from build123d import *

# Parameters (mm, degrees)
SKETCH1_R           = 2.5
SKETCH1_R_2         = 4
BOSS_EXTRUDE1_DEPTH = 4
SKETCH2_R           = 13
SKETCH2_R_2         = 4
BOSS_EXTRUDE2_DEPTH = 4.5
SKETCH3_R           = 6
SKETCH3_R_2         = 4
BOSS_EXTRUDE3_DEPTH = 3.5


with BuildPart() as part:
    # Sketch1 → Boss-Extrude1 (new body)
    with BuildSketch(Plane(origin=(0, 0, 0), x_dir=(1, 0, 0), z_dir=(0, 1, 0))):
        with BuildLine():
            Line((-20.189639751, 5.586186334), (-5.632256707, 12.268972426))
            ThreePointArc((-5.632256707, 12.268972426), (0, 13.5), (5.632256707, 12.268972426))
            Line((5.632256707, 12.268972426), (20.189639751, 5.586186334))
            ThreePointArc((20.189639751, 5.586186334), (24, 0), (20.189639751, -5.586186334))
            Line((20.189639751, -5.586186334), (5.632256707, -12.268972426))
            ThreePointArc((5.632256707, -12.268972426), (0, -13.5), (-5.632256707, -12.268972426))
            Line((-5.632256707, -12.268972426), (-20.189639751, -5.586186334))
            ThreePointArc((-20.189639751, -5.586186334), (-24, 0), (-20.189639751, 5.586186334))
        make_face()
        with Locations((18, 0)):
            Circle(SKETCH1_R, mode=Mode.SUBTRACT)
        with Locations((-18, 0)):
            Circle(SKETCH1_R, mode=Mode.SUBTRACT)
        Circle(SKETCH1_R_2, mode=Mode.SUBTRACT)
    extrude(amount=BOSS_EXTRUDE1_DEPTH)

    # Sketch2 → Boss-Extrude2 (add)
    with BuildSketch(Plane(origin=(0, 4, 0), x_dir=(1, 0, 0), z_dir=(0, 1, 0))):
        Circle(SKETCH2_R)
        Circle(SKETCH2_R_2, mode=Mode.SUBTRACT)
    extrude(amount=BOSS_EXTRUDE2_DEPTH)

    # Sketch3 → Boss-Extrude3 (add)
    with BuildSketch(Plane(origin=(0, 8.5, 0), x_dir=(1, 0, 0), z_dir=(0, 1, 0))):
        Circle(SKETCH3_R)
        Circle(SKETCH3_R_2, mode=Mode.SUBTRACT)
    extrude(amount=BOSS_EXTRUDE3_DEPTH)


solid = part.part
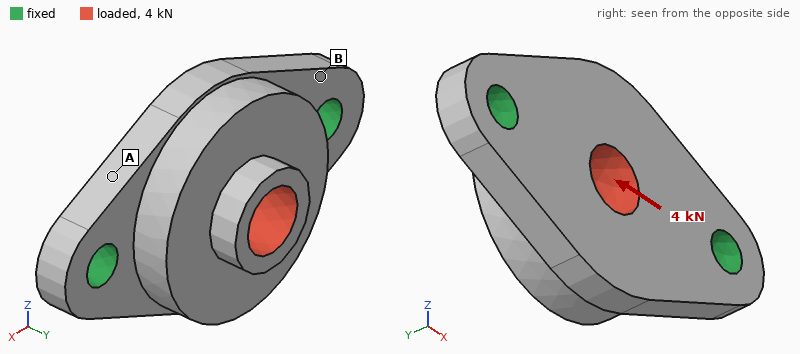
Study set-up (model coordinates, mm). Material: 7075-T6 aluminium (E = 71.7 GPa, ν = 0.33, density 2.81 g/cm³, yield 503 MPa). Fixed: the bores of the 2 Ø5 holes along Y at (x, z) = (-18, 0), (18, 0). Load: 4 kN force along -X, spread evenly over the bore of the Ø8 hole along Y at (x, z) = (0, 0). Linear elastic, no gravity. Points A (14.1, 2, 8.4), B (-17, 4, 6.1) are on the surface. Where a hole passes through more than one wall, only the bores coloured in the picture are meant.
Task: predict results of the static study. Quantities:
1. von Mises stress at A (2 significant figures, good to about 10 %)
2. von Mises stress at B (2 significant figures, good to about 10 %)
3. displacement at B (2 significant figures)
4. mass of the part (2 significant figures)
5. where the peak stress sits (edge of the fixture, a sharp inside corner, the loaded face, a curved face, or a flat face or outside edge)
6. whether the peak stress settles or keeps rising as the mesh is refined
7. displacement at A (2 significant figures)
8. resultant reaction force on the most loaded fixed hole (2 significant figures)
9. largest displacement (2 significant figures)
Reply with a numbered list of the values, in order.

1. 8.6 MPa
2. 15 MPa
3. 2.2 µm
4. 16 g
5. edge of the fixture
6. keeps rising
7. 4.3 µm
8. 2.1 kN
9. 13 µm
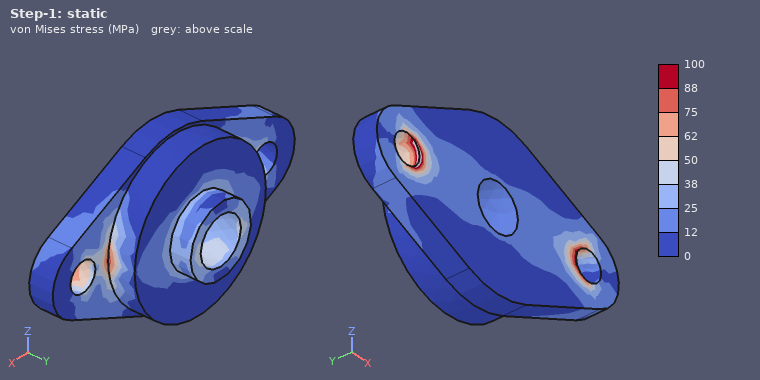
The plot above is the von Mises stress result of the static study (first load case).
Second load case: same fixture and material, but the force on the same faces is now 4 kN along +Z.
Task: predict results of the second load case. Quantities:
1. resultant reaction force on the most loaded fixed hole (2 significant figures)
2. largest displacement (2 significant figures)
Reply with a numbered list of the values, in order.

1. 2.0 kN
2. 74 µm
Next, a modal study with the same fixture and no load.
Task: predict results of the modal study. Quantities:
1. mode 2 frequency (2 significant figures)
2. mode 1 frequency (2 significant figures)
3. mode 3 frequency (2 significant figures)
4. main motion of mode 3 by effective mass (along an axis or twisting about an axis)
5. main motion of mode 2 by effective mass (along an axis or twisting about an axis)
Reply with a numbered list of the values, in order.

1. 16 kHz
2. 11 kHz
3. 27 kHz
4. along Z
5. along Y
